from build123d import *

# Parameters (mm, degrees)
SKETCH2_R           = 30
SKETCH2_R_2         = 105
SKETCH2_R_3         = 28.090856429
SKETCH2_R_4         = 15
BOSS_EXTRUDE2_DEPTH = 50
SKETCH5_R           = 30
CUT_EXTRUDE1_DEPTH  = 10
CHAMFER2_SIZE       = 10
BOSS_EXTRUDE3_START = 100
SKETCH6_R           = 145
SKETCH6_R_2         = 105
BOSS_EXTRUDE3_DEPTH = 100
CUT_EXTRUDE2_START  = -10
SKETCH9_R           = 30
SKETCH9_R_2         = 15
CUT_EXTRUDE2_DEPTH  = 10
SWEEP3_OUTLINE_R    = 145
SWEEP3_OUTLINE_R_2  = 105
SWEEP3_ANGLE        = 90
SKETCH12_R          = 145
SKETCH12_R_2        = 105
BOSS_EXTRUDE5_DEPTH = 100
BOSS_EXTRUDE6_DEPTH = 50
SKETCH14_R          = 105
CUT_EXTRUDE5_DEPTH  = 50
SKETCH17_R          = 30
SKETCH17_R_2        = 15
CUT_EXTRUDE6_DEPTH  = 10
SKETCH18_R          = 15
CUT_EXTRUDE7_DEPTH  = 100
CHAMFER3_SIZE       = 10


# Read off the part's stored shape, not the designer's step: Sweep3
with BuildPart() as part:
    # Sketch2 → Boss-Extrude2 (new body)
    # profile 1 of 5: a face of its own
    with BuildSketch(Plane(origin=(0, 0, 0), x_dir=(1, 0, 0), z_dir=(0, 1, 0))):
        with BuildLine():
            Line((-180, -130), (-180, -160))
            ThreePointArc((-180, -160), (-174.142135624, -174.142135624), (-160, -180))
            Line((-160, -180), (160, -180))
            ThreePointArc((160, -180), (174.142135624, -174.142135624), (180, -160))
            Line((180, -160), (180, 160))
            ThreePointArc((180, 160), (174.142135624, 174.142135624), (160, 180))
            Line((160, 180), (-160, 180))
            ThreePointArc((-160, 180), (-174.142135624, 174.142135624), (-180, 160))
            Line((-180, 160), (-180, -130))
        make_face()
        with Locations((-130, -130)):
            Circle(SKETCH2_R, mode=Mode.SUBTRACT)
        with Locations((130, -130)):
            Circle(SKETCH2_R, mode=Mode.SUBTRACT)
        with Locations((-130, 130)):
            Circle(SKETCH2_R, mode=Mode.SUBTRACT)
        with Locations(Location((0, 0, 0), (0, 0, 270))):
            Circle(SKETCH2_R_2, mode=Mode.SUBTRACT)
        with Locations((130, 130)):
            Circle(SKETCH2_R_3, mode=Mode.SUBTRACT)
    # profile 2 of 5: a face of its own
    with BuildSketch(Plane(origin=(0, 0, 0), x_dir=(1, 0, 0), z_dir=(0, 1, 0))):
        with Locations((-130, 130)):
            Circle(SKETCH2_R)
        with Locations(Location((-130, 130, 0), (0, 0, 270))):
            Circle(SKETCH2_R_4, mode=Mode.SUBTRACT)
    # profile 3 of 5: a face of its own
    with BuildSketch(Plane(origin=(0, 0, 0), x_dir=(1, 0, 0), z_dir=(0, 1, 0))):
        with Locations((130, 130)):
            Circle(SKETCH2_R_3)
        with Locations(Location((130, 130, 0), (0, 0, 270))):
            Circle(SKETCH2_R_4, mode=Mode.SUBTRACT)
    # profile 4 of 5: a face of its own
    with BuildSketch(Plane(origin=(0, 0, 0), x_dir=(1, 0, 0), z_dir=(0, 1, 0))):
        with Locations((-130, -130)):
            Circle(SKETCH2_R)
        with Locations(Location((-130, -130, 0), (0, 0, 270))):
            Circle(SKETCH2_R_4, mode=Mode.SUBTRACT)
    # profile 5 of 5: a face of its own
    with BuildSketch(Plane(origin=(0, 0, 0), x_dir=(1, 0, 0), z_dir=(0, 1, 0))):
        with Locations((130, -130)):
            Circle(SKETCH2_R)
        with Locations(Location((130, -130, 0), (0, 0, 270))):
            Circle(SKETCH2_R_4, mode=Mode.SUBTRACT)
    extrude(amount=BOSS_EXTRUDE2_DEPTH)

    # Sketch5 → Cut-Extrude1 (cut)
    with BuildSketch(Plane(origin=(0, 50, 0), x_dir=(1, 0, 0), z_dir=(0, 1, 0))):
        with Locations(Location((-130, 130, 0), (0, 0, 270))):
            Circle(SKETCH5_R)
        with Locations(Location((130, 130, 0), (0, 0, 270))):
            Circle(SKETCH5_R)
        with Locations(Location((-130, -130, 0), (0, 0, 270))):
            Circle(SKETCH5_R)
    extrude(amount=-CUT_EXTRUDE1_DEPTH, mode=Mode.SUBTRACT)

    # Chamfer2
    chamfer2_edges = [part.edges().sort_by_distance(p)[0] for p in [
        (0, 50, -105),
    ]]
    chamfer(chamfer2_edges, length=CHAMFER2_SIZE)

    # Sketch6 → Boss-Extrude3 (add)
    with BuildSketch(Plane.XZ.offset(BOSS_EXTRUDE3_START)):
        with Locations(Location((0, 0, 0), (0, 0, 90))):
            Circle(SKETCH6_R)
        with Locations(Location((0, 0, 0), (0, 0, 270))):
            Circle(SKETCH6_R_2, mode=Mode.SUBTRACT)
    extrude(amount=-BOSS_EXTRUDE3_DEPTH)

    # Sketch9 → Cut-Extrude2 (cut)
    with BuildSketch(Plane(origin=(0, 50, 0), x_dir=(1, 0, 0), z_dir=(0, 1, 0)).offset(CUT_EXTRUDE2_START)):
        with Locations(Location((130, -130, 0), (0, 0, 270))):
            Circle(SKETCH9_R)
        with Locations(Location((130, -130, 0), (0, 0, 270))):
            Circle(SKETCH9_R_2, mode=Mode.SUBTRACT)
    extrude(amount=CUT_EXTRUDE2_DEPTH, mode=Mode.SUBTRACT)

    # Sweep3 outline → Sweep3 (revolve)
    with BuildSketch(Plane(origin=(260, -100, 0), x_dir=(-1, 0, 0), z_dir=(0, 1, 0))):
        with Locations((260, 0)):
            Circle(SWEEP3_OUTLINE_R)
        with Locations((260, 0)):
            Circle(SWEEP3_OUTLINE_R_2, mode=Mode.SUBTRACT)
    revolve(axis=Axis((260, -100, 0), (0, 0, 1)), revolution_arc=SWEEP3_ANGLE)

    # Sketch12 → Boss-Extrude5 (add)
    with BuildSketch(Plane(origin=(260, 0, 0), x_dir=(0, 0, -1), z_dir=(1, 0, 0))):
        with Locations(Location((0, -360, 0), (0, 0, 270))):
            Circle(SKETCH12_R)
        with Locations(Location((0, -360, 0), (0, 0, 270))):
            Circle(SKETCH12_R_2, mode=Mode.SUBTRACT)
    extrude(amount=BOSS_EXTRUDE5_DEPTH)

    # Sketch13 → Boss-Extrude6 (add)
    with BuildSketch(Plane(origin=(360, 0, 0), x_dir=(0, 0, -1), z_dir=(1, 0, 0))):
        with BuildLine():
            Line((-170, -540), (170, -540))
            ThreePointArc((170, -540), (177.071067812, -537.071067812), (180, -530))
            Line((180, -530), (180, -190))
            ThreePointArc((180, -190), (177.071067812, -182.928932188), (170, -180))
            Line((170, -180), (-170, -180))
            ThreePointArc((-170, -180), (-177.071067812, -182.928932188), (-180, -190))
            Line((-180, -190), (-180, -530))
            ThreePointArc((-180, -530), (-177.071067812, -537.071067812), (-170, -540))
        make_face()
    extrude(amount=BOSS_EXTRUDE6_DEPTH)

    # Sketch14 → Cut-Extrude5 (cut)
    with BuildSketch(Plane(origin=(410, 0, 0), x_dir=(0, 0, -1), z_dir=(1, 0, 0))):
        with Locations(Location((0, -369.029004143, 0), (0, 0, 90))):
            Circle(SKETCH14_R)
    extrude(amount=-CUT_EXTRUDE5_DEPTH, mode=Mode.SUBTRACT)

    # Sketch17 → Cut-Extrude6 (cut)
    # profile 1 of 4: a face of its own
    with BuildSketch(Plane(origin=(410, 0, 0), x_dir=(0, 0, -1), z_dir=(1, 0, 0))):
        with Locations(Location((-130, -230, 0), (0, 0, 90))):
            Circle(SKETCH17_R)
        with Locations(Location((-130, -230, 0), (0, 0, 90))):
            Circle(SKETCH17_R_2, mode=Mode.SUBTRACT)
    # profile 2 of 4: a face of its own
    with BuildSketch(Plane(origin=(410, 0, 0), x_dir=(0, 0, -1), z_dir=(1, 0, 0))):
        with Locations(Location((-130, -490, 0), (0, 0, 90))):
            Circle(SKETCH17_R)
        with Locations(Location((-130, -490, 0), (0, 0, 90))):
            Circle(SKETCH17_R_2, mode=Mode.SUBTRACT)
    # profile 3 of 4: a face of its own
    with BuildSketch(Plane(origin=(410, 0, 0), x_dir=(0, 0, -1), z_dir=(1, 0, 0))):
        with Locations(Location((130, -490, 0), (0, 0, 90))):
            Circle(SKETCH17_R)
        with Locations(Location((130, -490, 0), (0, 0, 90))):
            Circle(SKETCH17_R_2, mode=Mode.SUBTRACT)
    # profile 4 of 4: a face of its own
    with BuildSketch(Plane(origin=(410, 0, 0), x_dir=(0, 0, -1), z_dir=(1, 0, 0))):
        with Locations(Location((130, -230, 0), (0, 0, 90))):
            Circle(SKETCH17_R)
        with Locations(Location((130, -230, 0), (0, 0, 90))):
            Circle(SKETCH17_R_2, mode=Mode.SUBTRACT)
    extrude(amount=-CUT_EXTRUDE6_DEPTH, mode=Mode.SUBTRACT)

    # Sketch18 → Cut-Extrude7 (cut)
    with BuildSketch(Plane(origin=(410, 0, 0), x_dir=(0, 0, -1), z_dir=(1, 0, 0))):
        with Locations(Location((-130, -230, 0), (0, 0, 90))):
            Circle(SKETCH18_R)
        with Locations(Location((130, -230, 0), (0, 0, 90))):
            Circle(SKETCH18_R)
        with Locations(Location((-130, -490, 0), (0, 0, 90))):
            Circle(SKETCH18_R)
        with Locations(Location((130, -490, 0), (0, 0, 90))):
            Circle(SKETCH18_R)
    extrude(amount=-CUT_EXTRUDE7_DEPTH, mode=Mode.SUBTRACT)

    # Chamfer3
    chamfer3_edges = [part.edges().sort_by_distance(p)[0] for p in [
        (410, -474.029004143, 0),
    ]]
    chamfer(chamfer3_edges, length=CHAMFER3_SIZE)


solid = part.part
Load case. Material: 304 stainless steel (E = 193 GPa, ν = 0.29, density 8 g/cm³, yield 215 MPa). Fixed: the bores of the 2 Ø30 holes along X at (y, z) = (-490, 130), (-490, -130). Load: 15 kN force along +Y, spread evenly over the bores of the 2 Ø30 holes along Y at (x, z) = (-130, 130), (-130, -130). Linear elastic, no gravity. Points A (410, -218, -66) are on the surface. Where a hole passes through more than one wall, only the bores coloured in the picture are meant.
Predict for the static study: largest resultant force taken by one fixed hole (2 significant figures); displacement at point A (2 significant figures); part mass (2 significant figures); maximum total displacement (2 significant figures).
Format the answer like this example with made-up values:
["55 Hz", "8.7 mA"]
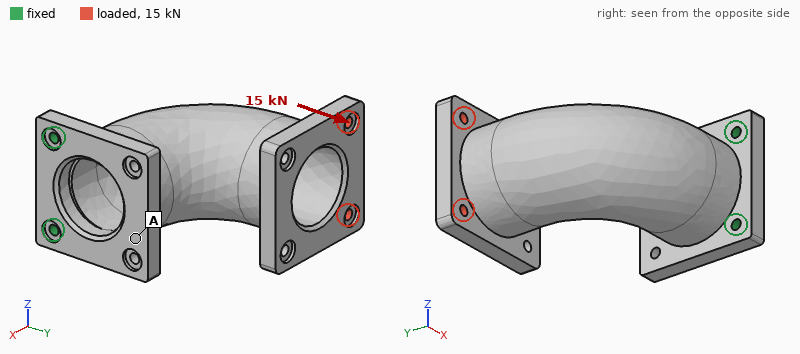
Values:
["7.5 kN", "0.28 mm", "220 kg", "0.88 mm"]
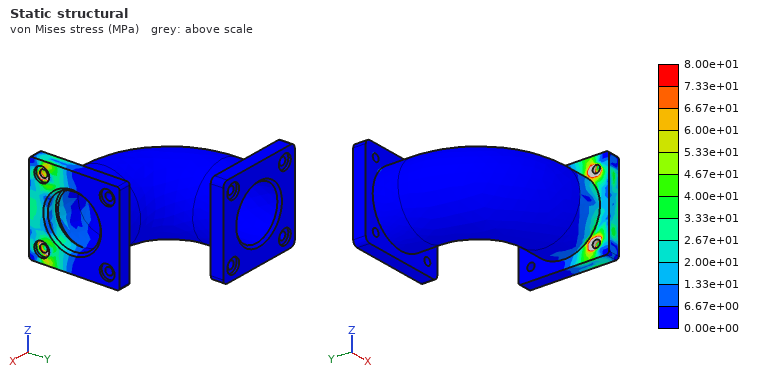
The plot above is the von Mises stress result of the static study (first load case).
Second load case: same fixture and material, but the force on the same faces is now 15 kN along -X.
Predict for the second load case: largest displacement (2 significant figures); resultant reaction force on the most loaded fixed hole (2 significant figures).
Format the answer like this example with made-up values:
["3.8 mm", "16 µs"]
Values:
["0.85 mm", "7.5 kN"]
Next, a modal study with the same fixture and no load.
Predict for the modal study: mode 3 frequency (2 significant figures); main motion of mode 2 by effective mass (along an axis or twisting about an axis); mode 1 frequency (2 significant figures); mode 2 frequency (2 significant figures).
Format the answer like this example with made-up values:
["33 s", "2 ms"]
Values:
["520 Hz", "along Z", "66 Hz", "210 Hz"]
